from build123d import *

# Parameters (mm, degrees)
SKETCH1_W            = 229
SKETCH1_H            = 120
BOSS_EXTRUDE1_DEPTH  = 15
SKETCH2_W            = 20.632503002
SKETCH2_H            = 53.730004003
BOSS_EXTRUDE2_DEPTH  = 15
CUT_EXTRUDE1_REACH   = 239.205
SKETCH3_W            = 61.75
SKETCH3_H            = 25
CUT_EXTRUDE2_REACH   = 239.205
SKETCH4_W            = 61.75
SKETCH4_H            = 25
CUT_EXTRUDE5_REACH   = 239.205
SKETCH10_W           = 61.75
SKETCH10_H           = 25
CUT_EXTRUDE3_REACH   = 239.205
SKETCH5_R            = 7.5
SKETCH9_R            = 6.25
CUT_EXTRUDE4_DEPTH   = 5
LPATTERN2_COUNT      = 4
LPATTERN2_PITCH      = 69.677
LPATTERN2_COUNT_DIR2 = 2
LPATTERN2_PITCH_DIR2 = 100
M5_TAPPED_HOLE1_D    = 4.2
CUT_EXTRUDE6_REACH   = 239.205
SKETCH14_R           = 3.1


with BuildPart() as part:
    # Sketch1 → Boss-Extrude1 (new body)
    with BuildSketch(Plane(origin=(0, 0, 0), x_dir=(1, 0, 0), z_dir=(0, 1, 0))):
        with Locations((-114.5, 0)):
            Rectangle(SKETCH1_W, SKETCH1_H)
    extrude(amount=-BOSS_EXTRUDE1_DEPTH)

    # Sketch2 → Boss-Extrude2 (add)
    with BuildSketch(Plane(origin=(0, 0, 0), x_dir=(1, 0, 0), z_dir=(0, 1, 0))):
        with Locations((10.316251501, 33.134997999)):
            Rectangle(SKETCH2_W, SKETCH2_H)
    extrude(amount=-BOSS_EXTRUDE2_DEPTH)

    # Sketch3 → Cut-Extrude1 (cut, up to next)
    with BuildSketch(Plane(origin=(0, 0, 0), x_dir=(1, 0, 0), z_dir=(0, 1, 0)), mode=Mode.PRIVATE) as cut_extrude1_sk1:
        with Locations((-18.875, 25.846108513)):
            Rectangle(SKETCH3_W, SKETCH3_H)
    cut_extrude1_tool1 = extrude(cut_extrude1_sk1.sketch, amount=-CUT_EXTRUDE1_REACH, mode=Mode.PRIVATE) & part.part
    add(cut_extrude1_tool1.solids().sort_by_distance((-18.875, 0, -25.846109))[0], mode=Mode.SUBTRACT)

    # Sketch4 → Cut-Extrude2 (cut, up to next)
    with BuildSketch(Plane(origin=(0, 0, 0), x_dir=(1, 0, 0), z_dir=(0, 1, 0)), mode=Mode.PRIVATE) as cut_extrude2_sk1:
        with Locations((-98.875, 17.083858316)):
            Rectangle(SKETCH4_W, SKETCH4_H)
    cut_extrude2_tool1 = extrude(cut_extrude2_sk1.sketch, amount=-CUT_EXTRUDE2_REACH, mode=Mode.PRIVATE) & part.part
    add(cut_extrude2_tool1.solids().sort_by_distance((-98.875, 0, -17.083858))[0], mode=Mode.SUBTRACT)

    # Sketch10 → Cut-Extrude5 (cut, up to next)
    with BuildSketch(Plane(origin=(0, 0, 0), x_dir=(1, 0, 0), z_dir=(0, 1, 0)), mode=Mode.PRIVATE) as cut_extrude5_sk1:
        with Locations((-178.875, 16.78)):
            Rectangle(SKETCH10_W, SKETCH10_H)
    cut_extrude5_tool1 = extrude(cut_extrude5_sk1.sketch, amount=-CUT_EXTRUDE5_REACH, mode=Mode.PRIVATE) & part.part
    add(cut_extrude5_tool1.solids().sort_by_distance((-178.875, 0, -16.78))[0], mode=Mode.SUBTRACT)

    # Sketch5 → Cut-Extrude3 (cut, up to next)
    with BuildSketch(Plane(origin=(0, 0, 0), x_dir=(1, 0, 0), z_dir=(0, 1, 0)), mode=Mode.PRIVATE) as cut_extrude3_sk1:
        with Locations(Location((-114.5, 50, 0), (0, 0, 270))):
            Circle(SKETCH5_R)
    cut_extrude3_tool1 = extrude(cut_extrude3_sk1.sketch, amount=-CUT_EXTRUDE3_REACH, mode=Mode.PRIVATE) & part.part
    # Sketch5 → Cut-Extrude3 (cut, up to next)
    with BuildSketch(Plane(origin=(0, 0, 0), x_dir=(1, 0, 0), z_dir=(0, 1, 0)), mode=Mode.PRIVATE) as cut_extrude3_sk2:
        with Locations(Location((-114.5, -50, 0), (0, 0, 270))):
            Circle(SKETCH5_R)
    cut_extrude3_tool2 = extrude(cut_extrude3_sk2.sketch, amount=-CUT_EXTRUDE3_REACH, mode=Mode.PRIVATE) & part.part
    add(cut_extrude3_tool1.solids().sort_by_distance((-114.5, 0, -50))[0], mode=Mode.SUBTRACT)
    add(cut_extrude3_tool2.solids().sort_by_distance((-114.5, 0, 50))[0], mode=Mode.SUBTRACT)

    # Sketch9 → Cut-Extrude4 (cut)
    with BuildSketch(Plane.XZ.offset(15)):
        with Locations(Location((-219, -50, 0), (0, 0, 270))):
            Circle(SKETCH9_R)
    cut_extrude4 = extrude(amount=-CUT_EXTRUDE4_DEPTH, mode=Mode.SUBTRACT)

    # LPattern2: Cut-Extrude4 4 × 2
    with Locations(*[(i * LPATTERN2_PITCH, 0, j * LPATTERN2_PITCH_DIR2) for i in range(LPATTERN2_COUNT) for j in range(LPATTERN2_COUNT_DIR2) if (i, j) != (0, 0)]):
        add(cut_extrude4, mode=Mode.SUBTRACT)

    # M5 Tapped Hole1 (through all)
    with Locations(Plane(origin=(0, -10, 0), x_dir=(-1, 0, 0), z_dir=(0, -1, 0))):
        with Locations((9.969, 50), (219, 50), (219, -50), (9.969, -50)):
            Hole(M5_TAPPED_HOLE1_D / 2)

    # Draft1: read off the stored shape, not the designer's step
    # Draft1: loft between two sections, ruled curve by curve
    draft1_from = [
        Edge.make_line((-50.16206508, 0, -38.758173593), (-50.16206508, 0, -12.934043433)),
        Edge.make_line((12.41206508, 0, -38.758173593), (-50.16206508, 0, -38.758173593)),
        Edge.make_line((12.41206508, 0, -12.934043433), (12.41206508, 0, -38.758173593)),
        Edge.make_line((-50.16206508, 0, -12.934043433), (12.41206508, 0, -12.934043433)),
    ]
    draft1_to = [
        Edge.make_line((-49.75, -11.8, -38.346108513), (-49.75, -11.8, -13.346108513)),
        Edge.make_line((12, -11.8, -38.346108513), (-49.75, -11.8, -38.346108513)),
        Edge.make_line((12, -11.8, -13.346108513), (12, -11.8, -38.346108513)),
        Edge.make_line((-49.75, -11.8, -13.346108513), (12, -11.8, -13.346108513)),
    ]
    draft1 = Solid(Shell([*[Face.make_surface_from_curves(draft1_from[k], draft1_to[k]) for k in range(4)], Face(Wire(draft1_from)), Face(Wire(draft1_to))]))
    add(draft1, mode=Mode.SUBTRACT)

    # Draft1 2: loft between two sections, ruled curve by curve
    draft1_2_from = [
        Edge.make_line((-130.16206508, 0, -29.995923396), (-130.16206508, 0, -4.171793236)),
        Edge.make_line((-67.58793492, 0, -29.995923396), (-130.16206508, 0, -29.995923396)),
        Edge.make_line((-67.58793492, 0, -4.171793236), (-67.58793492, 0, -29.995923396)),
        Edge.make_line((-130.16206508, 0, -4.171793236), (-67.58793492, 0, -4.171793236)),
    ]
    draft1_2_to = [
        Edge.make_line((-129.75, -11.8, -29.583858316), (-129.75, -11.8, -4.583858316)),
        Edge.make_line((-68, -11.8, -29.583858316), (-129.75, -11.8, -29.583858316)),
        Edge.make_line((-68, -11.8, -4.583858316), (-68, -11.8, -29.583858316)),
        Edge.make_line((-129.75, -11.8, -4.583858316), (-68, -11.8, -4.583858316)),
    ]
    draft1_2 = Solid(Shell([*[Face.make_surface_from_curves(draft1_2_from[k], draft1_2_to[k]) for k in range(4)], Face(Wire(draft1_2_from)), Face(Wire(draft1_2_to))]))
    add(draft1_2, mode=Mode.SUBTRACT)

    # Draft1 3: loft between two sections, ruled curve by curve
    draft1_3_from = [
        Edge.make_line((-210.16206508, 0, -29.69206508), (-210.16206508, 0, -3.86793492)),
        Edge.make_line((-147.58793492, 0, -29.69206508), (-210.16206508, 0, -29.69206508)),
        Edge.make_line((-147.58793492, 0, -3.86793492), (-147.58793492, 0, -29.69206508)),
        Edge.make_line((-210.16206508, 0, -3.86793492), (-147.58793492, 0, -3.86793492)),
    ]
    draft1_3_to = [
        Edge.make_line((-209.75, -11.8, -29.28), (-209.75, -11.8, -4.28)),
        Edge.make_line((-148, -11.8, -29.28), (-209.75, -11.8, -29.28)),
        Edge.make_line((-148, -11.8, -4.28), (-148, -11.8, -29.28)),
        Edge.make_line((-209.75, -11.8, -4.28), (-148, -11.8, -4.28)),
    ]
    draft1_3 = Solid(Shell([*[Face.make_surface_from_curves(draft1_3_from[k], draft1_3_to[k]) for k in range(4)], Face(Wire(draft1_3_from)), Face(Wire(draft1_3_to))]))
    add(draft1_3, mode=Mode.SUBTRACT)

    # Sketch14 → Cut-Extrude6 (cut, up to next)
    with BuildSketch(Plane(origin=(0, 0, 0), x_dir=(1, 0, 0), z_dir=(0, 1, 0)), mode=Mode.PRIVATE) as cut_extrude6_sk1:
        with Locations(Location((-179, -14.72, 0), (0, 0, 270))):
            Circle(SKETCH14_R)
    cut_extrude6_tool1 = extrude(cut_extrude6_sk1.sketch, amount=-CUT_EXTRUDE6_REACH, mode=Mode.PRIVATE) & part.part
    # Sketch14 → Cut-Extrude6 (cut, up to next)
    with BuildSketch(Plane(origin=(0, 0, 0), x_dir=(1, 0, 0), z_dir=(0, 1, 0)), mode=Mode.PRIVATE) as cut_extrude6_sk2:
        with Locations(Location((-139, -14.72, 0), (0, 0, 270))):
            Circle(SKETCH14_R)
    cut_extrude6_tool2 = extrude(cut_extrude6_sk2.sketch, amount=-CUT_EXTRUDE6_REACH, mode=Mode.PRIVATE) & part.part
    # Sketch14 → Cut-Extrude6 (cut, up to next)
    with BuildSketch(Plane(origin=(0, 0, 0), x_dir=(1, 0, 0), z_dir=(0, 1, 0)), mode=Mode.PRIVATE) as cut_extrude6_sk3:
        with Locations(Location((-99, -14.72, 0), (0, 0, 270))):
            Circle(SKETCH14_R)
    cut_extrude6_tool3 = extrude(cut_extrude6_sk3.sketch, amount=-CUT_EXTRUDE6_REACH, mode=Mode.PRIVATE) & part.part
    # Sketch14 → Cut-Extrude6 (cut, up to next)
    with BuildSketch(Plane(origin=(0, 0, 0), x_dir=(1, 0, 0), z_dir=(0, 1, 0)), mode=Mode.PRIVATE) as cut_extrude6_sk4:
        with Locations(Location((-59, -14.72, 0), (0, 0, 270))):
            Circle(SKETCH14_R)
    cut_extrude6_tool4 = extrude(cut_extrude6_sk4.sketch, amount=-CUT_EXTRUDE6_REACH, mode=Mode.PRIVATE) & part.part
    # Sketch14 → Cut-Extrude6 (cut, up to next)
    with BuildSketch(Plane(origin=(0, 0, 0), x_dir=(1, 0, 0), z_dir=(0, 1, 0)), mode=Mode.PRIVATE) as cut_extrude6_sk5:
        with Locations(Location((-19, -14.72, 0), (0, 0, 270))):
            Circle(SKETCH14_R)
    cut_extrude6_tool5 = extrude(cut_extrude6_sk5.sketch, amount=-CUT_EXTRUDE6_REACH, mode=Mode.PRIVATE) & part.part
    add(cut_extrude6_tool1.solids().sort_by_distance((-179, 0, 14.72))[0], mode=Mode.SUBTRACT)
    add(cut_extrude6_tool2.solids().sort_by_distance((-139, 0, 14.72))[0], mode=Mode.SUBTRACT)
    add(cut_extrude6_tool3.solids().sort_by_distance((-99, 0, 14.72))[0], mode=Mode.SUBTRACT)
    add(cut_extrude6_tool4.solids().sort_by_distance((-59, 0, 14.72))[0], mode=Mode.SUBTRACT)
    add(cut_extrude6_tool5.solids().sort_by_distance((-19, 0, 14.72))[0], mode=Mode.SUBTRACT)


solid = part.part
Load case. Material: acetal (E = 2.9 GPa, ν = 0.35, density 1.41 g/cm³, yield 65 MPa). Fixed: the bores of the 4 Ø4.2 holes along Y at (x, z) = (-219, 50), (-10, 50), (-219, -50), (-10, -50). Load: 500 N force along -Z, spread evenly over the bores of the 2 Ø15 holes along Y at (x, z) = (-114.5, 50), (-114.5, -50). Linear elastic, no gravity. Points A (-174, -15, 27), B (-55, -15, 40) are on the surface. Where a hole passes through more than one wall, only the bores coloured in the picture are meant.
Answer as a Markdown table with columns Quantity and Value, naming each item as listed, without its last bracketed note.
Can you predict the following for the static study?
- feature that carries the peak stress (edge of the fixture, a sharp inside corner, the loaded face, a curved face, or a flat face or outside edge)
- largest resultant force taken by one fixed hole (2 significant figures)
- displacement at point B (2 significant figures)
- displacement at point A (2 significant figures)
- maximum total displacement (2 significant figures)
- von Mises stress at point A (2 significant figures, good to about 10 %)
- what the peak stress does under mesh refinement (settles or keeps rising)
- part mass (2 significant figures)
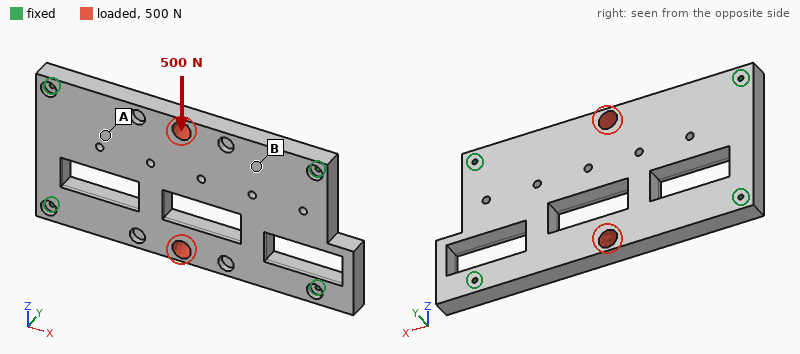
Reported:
| Quantity | Value |
|---|---|
| feature that carries the peak stress | edge of the fixture |
| largest resultant force taken by one fixed hole | 280 N |
| displacement at point B | 29 µm |
| displacement at point A | 29 µm |
| maximum total displacement | 68 µm |
| von Mises stress at point A | 0.53 MPa |
| what the peak stress does under mesh refinement | keeps rising |
| part mass | 490 g |
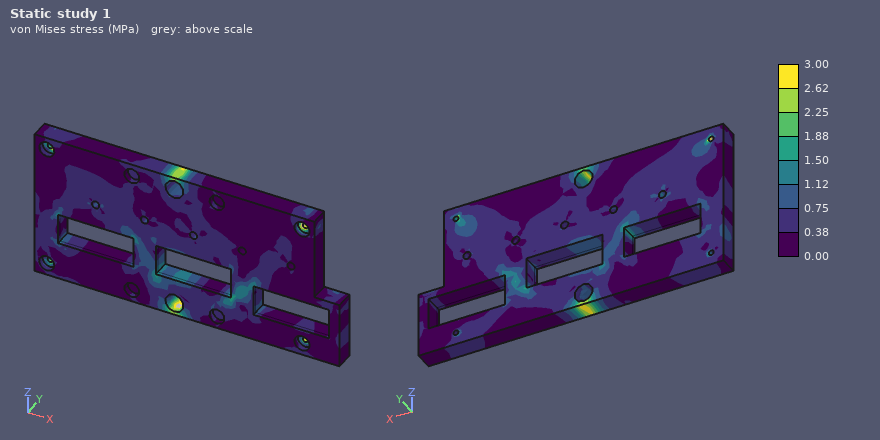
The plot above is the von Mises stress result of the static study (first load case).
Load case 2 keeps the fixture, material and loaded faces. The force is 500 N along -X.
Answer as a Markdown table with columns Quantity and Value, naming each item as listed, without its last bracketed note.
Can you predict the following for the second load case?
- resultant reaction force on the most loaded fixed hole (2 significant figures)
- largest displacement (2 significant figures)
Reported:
| Quantity | Value |
|---|---|
| resultant reaction force on the most loaded fixed hole | 130 N |
| largest displacement | 15 µm |
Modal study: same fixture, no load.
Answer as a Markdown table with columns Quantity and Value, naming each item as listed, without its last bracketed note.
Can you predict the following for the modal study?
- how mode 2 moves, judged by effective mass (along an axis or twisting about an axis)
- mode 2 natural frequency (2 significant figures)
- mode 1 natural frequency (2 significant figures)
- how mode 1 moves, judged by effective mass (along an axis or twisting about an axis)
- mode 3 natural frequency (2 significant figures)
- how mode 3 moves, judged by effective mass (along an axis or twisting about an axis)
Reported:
| Quantity | Value |
|---|---|
| how mode 2 moves, judged by effective mass | twisting about X |
| mode 2 natural frequency | 560 Hz |
| mode 1 natural frequency | 320 Hz |
| how mode 1 moves, judged by effective mass | along Y |
| mode 3 natural frequency | 850 Hz |
| how mode 3 moves, judged by effective mass | twisting about Z |
